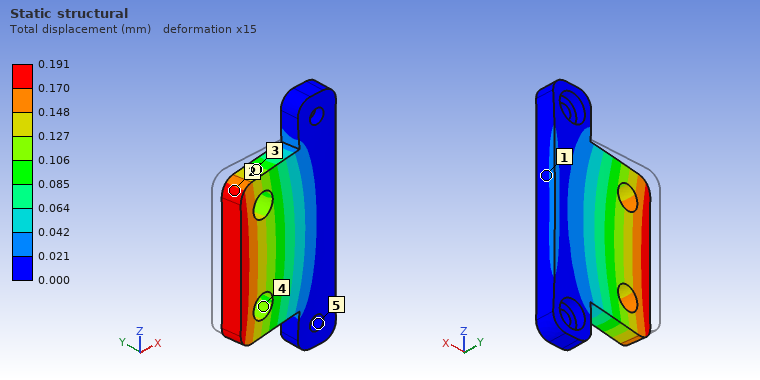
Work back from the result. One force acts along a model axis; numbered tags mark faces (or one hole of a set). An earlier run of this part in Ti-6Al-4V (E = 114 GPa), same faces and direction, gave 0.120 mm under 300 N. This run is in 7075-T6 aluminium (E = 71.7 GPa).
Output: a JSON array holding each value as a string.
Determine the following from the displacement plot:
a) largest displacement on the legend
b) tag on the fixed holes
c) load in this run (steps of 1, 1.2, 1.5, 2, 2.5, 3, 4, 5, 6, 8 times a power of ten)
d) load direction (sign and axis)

["0.191 mm", "5", "300 N", "-Y"]
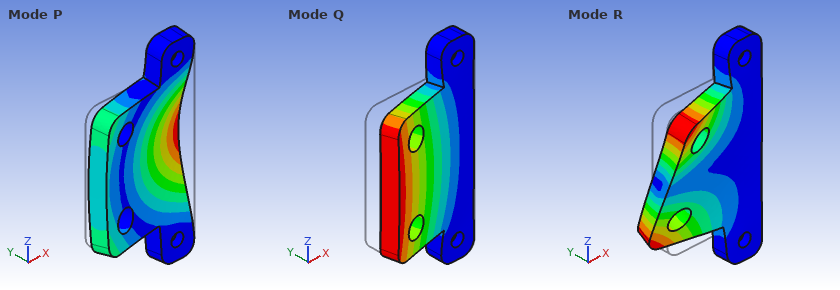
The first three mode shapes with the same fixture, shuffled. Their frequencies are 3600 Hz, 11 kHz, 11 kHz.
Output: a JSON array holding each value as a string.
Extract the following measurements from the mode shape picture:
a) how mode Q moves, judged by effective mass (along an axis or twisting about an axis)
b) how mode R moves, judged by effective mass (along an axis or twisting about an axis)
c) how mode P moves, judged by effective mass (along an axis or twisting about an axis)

["along Y", "twisting about X", "along Y"]
